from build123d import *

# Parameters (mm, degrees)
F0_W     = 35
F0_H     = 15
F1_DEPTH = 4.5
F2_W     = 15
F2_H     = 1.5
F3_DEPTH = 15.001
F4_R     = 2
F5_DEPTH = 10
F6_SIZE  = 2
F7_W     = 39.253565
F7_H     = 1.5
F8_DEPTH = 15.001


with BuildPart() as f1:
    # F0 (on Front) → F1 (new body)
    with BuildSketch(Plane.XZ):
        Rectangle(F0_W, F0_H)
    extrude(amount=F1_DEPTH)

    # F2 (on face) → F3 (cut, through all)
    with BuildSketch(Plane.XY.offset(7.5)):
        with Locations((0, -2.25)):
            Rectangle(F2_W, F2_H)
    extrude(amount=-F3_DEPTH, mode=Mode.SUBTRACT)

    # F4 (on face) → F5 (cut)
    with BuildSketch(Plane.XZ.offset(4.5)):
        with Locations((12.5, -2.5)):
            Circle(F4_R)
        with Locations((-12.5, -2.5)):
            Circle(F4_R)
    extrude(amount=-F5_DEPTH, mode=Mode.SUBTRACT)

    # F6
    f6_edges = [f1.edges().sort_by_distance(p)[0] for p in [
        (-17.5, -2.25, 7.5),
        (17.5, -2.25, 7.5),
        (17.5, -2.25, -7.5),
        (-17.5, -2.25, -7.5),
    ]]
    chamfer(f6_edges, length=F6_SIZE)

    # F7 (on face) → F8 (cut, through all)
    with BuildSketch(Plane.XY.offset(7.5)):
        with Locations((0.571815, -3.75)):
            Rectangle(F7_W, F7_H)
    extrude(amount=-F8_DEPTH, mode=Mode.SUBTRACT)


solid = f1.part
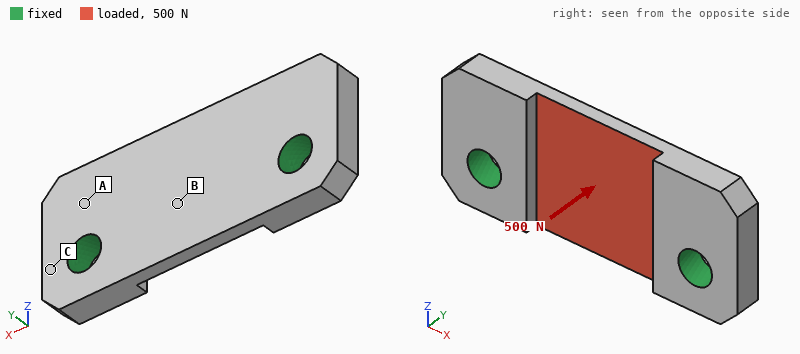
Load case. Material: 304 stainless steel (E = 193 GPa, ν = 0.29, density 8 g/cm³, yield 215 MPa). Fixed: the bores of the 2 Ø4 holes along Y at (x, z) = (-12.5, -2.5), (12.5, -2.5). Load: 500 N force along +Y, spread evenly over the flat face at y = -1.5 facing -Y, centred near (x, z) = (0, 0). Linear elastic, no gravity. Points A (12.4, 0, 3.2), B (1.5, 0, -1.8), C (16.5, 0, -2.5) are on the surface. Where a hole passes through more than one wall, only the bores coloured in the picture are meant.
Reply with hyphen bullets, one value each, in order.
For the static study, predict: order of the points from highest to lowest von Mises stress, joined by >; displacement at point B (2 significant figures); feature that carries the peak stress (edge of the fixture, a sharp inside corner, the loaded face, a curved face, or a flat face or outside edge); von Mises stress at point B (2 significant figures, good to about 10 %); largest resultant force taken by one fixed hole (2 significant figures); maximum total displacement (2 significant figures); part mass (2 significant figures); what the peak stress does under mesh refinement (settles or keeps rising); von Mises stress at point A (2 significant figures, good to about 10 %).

- B > A > C
- 11 µm
- edge of the fixture
- 71 MPa
- 300 N
- 18 µm
- 9.1 g
- keeps rising
- 30 MPa
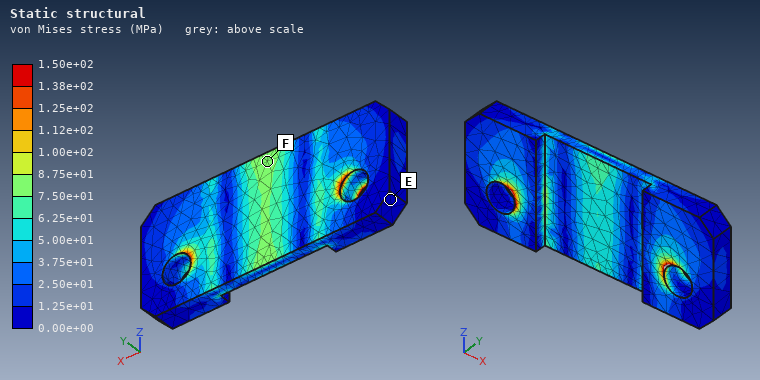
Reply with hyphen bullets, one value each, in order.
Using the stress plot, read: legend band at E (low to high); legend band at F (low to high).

- 0.00e+00 to 1.25e+01 MPa
- 7.50e+01 to 8.75e+01 MPa
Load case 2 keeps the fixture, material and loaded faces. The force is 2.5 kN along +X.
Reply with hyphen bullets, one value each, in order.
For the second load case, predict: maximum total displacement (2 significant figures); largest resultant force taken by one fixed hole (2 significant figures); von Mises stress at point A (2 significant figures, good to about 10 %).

- 5.2 µm
- 1.3 kN
- 37 MPa
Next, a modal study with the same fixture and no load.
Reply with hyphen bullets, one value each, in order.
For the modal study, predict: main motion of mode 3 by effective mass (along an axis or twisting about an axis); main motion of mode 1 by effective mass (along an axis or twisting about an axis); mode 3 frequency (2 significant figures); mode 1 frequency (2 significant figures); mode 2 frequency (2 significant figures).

- twisting about Z
- along Y
- 28 kHz
- 19 kHz
- 25 kHz
